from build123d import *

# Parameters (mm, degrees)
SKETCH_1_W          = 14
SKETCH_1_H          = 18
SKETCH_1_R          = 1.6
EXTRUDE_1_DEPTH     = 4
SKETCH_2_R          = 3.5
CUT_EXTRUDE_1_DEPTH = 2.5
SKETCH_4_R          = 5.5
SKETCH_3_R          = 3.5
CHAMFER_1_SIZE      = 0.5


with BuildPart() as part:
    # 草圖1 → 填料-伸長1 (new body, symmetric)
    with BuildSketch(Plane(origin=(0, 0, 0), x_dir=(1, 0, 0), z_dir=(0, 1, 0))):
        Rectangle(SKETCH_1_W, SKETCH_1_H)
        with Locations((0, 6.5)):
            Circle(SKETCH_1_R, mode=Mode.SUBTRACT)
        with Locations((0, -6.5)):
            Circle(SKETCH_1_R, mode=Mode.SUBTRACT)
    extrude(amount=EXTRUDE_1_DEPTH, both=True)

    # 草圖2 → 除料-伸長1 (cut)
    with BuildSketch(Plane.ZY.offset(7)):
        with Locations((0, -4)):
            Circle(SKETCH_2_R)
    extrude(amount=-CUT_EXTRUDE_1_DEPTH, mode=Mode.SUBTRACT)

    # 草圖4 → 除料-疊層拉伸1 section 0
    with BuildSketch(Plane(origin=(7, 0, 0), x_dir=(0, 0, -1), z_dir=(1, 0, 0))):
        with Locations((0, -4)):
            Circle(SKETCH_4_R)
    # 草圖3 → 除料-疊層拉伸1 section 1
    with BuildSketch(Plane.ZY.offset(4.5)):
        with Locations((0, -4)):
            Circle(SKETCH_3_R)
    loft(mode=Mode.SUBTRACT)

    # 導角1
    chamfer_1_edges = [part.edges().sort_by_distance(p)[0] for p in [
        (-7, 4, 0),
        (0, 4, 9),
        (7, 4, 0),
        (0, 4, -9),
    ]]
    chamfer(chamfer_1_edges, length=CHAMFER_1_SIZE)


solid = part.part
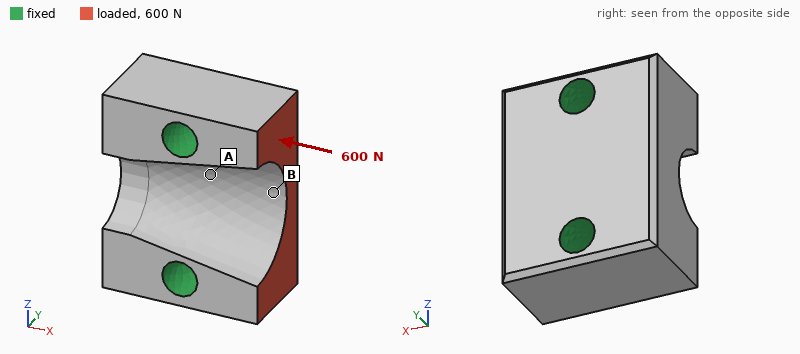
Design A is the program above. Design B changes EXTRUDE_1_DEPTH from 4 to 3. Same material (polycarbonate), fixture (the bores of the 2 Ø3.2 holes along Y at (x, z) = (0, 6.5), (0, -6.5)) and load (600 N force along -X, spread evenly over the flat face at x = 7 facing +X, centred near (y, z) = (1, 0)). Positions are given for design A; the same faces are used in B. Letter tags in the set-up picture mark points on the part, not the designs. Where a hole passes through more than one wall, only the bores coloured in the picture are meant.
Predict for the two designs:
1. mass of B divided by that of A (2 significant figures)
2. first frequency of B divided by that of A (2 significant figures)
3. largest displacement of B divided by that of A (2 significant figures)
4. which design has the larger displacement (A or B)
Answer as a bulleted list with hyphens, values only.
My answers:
- 0.76
- 0.90
- 1.4
- B
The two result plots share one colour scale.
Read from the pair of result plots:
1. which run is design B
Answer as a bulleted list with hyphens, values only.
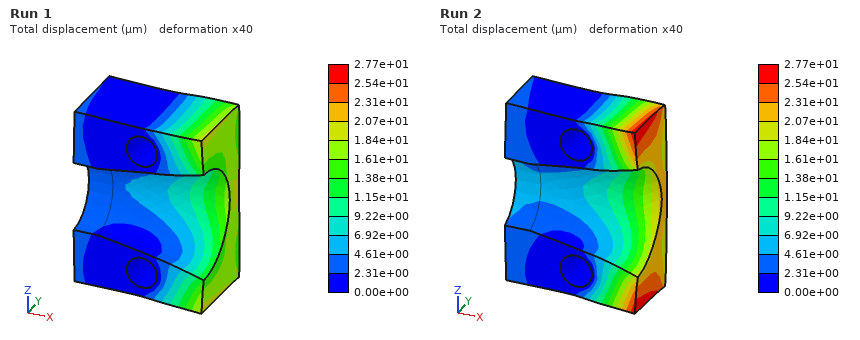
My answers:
- Run 2
